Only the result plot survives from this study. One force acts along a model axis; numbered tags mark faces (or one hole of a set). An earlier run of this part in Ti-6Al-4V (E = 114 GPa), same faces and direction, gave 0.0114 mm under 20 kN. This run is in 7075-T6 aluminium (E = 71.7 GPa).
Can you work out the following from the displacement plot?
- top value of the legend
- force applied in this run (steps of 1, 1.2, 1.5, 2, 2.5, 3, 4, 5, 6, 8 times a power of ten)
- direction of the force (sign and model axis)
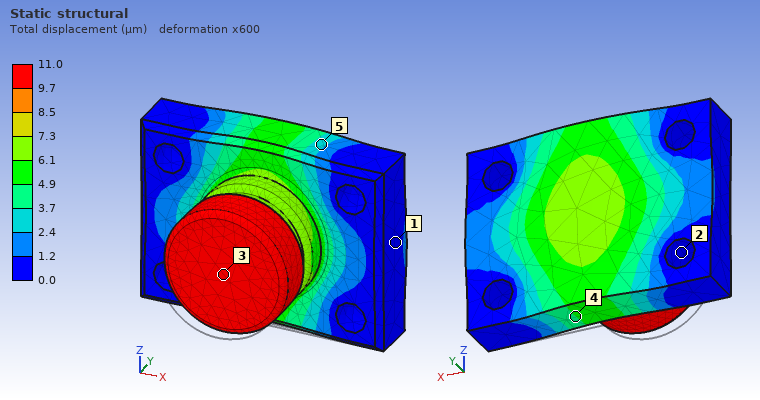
11.0 µm
12 kN
+Y
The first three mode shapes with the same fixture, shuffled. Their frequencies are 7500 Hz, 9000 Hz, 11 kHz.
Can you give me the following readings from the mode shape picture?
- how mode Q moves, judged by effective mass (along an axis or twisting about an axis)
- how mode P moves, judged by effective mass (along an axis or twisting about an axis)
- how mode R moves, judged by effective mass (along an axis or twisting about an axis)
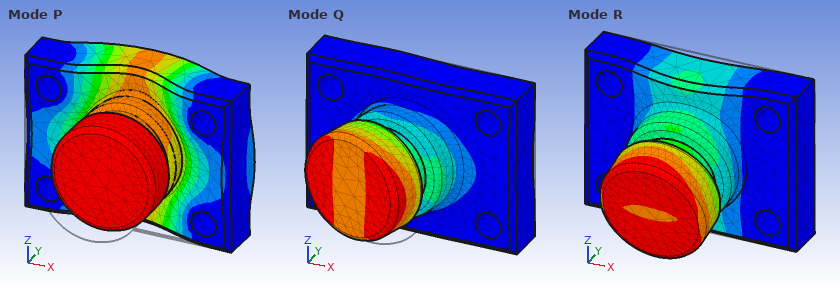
along X
along Y
along Z
